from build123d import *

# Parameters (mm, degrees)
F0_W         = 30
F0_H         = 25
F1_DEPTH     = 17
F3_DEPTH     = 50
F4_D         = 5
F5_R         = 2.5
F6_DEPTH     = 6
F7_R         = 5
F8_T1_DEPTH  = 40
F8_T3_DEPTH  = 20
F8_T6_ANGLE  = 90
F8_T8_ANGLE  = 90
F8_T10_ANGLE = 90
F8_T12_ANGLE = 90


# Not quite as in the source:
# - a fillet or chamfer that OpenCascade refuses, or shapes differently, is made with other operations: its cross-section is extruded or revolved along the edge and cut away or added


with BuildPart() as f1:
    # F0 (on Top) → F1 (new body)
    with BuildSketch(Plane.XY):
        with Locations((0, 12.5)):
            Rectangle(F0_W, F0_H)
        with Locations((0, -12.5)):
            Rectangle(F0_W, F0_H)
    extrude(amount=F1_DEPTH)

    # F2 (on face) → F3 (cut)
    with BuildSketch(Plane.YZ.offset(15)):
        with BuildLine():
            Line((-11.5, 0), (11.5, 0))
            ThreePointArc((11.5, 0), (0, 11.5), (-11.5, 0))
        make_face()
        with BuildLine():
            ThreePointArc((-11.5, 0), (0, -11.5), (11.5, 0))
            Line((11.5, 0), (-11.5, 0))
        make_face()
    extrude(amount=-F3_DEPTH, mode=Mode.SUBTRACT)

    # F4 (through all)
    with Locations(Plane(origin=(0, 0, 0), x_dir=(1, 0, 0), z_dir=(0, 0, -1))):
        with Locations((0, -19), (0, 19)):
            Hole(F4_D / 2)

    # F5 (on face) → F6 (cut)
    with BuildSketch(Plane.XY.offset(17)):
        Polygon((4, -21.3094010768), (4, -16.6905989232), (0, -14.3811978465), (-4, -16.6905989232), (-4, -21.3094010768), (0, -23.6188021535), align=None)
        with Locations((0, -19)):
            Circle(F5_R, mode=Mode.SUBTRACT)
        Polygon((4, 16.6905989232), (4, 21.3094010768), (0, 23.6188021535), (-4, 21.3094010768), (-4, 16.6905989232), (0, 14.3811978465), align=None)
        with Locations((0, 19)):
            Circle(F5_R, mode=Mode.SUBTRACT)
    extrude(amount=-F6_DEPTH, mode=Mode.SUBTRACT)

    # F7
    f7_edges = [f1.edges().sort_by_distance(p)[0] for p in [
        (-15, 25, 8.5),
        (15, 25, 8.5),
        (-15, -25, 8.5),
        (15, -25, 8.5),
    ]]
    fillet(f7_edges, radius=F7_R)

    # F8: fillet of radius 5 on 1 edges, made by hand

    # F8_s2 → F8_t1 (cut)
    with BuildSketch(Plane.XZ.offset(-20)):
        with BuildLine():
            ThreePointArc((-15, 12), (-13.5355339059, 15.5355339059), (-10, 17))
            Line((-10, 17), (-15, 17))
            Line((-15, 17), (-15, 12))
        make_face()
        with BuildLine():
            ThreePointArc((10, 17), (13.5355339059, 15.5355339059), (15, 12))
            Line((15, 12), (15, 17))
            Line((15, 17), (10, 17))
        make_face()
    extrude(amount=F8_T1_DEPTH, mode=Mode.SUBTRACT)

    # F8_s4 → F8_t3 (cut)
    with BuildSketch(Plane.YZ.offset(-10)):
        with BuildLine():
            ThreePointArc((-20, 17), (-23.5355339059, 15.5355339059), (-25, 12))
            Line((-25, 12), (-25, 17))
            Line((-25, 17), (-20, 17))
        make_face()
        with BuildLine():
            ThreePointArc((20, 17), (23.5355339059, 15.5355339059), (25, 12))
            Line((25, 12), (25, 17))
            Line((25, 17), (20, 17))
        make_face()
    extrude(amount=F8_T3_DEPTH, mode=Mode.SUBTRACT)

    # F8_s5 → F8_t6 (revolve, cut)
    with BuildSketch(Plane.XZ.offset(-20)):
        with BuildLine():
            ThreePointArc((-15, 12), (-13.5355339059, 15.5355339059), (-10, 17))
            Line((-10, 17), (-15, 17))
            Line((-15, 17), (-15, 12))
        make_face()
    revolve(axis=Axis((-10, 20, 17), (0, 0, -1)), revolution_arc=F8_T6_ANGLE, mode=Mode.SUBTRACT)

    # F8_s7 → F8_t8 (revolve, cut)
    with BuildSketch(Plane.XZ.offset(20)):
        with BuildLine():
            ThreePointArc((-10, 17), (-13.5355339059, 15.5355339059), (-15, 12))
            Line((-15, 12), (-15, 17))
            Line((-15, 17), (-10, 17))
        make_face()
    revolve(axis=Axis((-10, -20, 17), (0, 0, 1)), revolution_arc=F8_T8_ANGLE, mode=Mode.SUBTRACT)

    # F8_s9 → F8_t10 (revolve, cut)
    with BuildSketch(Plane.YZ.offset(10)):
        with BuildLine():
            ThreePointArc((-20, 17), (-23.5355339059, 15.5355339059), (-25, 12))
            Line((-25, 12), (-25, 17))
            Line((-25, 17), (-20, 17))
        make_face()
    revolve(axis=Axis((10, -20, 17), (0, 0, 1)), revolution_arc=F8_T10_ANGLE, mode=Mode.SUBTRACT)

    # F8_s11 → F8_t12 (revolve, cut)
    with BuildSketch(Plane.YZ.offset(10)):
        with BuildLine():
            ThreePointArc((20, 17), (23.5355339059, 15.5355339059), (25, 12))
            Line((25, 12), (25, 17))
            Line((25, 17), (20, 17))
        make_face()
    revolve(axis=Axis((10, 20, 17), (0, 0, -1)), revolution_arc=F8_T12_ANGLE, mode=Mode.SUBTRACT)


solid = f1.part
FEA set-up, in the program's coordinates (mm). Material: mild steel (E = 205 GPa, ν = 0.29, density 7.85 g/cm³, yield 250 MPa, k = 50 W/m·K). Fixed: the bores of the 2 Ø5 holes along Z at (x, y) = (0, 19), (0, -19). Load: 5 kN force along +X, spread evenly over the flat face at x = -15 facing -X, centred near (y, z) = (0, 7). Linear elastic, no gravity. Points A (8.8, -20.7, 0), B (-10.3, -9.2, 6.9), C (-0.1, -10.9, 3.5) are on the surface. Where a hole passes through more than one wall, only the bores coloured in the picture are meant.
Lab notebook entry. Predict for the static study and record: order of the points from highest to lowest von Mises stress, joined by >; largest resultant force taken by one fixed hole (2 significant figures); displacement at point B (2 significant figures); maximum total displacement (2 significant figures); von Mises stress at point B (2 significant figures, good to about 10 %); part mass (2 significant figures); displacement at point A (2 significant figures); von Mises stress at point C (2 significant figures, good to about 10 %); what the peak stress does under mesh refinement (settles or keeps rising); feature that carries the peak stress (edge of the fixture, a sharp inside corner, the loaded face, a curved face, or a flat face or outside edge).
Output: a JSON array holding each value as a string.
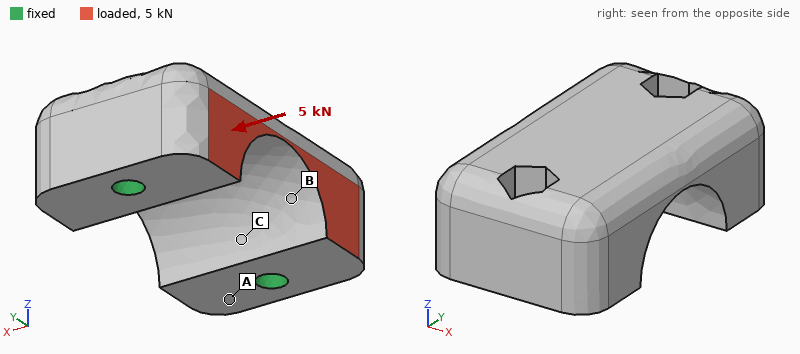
["B > C > A", "2.5 kN", "1.9 µm", "2.4 µm", "18 MPa", "130 g", "0.49 µm", "10 MPa", "keeps rising", "edge of the fixture"]
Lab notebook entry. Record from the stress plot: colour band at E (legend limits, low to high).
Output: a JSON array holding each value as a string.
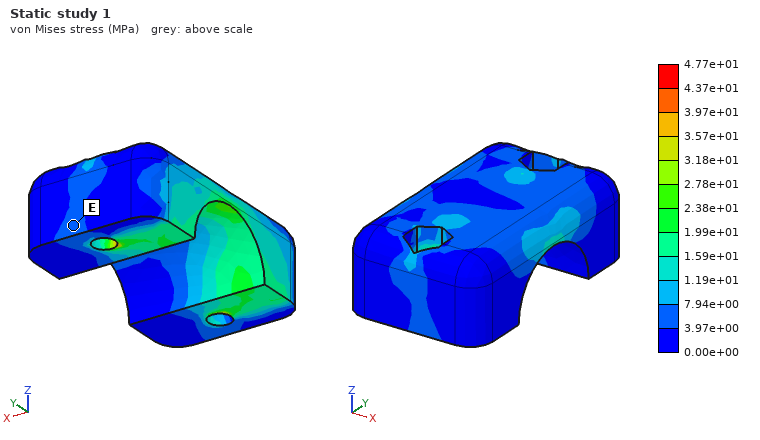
["3.97e+00 to 7.94e+00 MPa"]
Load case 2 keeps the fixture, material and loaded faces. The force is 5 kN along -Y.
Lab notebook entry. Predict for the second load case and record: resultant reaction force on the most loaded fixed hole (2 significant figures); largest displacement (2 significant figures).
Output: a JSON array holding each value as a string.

["2.9 kN", "6.9 µm"]
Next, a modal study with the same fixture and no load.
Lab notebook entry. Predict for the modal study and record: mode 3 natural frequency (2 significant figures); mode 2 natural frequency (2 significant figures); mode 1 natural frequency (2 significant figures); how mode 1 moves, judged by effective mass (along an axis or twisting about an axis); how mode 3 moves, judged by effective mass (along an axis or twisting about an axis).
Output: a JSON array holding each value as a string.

["27 kHz", "25 kHz", "18 kHz", "along X", "along Z"]
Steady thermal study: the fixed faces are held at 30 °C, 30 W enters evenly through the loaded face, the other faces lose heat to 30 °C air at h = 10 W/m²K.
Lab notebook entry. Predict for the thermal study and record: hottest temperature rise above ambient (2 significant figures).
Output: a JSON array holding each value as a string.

["24 K"]
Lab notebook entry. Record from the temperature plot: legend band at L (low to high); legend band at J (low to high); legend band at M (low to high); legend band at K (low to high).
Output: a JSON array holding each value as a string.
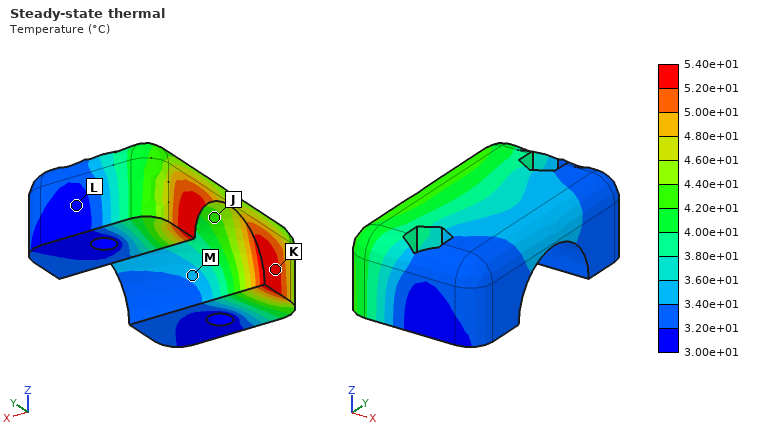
["3.00e+01 to 3.20e+01 °C", "4.20e+01 to 4.40e+01 °C", "3.40e+01 to 3.60e+01 °C", "5.20e+01 to 5.40e+01 °C"]
